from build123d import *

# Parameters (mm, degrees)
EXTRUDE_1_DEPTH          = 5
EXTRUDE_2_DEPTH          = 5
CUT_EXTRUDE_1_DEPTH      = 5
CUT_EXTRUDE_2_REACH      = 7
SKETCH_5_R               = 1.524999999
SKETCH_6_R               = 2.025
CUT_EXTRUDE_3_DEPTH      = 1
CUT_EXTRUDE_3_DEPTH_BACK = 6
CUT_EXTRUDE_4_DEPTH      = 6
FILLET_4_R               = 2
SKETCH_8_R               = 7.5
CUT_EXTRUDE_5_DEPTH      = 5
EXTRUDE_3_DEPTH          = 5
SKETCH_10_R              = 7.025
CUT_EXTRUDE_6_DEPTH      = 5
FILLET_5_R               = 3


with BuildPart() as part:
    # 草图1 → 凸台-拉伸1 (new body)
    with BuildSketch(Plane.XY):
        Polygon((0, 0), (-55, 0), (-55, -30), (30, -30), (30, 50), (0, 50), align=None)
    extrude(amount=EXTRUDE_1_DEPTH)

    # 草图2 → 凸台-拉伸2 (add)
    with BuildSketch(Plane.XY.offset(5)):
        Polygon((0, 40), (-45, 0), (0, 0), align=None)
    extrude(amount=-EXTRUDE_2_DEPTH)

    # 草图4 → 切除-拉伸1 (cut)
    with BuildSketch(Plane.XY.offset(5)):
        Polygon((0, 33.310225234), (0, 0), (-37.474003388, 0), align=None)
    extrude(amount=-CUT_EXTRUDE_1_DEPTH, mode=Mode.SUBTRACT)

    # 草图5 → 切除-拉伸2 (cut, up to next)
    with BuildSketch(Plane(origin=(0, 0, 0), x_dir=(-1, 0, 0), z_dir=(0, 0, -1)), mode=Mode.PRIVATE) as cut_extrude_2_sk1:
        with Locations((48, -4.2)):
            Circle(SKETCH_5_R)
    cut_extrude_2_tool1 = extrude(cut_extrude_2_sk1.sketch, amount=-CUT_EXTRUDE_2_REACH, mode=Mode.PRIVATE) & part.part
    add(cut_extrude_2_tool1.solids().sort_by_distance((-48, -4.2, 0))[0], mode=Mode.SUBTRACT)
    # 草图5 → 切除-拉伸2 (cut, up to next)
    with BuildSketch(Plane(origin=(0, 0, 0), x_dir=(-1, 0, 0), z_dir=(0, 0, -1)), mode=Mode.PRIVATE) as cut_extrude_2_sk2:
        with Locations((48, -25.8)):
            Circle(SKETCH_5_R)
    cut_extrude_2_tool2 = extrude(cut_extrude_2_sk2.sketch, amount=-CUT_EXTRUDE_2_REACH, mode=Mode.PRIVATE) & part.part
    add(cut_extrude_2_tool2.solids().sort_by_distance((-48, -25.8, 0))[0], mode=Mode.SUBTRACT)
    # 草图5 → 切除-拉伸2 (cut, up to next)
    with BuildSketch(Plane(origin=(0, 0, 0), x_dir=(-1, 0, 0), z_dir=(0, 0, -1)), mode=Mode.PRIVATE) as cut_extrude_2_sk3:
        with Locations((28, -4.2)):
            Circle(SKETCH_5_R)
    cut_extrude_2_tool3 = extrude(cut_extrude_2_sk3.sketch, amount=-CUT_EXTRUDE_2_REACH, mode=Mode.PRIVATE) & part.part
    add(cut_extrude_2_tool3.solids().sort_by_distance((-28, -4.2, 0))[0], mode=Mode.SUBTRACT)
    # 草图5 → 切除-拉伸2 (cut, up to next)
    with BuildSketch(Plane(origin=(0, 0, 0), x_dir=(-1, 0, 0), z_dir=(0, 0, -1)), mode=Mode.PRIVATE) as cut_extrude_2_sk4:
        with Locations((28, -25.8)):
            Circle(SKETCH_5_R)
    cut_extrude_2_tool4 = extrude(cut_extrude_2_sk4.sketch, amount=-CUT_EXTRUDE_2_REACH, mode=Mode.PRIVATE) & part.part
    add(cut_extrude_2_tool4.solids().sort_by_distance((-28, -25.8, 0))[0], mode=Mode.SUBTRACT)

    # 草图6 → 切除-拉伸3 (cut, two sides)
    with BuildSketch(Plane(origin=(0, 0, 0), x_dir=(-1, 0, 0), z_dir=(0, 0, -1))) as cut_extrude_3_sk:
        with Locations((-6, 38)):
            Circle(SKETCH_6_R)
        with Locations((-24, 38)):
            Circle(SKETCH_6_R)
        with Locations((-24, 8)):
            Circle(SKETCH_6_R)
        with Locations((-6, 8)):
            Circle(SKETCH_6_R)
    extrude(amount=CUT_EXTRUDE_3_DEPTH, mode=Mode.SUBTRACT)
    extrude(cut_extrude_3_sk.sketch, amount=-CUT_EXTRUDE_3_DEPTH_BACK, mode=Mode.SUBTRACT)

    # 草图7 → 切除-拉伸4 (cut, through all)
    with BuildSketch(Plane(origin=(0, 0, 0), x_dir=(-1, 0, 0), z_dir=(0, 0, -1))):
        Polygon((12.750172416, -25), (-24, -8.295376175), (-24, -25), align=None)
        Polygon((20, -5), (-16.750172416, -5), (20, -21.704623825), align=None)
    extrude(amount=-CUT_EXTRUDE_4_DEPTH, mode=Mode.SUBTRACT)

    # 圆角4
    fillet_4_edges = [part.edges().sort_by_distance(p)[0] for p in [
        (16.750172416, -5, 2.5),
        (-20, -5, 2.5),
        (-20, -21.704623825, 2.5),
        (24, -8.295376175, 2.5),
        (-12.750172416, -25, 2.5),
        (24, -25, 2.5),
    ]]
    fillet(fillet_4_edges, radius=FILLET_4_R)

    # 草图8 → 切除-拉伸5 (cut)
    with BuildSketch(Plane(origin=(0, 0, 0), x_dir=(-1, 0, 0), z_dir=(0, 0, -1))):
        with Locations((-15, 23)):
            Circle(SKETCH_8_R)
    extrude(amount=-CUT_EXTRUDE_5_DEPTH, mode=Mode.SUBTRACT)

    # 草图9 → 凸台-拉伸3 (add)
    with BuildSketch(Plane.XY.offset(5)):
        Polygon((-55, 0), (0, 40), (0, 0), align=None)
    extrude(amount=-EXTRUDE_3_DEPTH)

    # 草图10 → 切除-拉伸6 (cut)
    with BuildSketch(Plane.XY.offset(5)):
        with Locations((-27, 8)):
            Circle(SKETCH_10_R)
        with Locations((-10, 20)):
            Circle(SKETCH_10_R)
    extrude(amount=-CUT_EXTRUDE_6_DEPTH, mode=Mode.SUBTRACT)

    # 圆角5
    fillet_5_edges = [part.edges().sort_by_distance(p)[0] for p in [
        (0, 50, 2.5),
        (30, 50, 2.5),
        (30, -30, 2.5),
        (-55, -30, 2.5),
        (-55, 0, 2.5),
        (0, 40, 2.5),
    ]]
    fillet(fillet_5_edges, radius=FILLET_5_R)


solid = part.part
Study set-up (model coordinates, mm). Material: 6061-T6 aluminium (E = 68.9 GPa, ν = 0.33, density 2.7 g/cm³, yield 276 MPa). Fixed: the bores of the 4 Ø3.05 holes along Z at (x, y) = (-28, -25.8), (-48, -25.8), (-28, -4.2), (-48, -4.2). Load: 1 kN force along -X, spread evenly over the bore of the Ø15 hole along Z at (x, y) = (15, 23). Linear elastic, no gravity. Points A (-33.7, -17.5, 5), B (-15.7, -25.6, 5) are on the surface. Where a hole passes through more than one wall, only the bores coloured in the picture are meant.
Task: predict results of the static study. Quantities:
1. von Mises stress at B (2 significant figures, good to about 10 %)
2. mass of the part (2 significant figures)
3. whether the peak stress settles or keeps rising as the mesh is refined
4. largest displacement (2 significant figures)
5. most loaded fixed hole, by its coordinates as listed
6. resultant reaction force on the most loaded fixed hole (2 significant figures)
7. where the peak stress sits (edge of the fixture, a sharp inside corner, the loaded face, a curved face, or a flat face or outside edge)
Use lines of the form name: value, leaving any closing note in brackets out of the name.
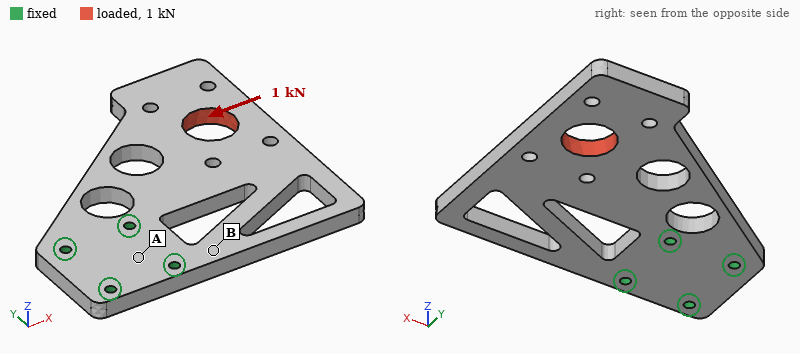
von Mises stress at B: 14 MPa
mass of the part: 54 g
whether the peak stress settles or keeps rising as the mesh is refined: keeps rising
largest displacement: 74 µm
most loaded fixed hole, by its coordinates as listed: (-28, -4.2)
resultant reaction force on the most loaded fixed hole: 1.2 kN
where the peak stress sits: edge of the fixture
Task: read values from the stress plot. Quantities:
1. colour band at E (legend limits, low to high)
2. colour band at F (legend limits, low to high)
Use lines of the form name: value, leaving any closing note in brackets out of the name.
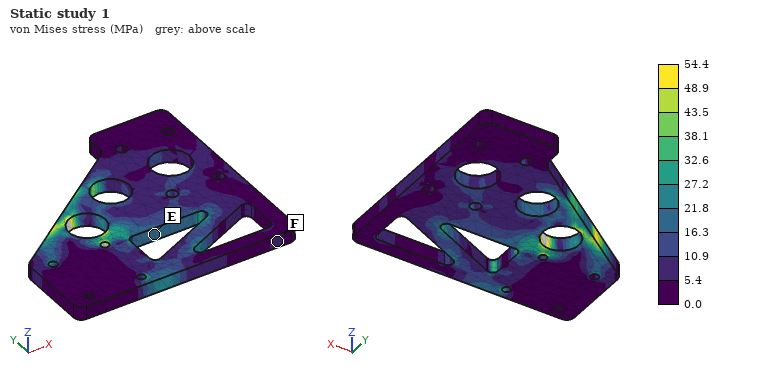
colour band at E: 16.3 to 21.8 MPa
colour band at F: 5.4 to 10.9 MPa
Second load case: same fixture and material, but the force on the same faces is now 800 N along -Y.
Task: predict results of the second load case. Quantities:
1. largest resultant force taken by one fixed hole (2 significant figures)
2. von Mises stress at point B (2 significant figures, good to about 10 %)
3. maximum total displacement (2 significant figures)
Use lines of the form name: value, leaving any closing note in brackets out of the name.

largest resultant force taken by one fixed hole: 1.1 kN
von Mises stress at point B: 22 MPa
maximum total displacement: 85 µm
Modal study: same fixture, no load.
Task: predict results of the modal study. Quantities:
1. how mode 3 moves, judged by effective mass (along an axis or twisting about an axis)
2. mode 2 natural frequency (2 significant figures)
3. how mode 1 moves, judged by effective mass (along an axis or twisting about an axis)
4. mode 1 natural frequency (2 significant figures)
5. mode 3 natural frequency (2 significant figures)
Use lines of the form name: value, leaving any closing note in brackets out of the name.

how mode 3 moves, judged by effective mass: along Y
mode 2 natural frequency: 1400 Hz
how mode 1 moves, judged by effective mass: along Z
mode 1 natural frequency: 610 Hz
mode 3 natural frequency: 3200 Hz
